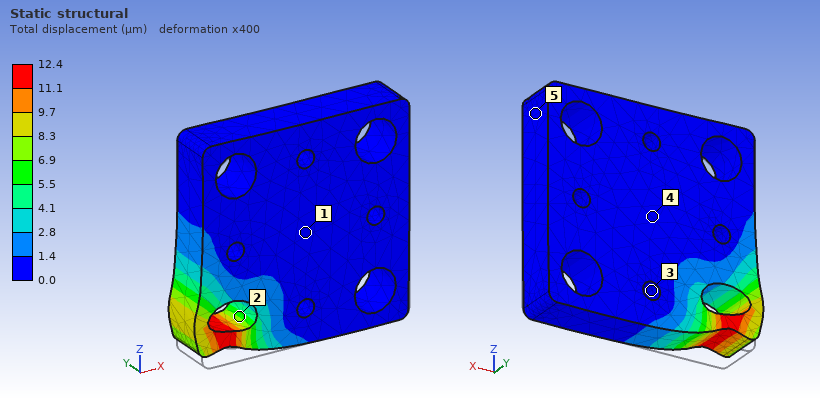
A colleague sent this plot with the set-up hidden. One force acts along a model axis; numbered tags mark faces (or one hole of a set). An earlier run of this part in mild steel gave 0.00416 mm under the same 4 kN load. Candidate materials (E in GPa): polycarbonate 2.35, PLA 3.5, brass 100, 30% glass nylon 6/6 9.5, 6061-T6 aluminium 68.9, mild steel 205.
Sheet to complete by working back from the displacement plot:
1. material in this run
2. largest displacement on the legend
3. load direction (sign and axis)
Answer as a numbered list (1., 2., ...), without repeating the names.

1. 6061-T6 aluminium
2. 12.4 µm
3. +Z
